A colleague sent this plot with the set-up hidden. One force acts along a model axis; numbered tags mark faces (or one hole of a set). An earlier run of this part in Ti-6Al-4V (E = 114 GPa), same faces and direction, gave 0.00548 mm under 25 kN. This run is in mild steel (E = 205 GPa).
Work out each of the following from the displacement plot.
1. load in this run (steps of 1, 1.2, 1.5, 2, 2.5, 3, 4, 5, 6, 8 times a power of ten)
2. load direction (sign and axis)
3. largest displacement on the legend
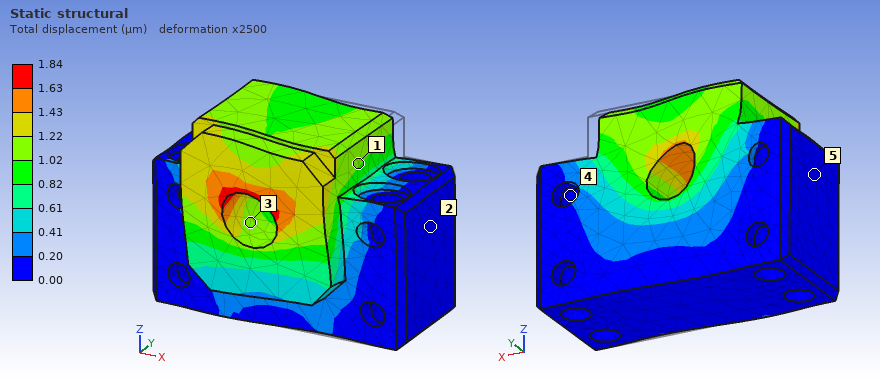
15 kN
-X
1.84 µm
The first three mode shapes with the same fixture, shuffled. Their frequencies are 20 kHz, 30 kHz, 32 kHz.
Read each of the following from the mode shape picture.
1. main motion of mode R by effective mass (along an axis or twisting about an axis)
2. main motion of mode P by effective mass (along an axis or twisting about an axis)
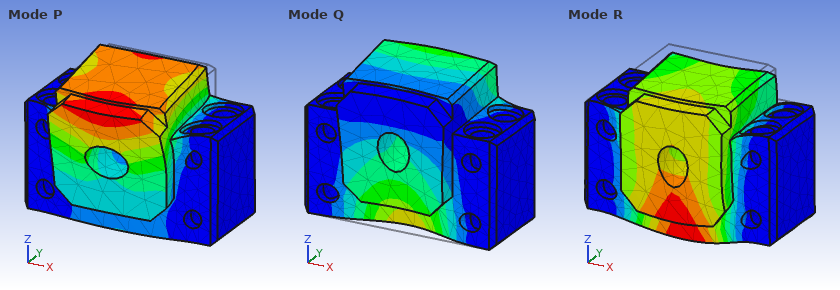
along Z
along Y
